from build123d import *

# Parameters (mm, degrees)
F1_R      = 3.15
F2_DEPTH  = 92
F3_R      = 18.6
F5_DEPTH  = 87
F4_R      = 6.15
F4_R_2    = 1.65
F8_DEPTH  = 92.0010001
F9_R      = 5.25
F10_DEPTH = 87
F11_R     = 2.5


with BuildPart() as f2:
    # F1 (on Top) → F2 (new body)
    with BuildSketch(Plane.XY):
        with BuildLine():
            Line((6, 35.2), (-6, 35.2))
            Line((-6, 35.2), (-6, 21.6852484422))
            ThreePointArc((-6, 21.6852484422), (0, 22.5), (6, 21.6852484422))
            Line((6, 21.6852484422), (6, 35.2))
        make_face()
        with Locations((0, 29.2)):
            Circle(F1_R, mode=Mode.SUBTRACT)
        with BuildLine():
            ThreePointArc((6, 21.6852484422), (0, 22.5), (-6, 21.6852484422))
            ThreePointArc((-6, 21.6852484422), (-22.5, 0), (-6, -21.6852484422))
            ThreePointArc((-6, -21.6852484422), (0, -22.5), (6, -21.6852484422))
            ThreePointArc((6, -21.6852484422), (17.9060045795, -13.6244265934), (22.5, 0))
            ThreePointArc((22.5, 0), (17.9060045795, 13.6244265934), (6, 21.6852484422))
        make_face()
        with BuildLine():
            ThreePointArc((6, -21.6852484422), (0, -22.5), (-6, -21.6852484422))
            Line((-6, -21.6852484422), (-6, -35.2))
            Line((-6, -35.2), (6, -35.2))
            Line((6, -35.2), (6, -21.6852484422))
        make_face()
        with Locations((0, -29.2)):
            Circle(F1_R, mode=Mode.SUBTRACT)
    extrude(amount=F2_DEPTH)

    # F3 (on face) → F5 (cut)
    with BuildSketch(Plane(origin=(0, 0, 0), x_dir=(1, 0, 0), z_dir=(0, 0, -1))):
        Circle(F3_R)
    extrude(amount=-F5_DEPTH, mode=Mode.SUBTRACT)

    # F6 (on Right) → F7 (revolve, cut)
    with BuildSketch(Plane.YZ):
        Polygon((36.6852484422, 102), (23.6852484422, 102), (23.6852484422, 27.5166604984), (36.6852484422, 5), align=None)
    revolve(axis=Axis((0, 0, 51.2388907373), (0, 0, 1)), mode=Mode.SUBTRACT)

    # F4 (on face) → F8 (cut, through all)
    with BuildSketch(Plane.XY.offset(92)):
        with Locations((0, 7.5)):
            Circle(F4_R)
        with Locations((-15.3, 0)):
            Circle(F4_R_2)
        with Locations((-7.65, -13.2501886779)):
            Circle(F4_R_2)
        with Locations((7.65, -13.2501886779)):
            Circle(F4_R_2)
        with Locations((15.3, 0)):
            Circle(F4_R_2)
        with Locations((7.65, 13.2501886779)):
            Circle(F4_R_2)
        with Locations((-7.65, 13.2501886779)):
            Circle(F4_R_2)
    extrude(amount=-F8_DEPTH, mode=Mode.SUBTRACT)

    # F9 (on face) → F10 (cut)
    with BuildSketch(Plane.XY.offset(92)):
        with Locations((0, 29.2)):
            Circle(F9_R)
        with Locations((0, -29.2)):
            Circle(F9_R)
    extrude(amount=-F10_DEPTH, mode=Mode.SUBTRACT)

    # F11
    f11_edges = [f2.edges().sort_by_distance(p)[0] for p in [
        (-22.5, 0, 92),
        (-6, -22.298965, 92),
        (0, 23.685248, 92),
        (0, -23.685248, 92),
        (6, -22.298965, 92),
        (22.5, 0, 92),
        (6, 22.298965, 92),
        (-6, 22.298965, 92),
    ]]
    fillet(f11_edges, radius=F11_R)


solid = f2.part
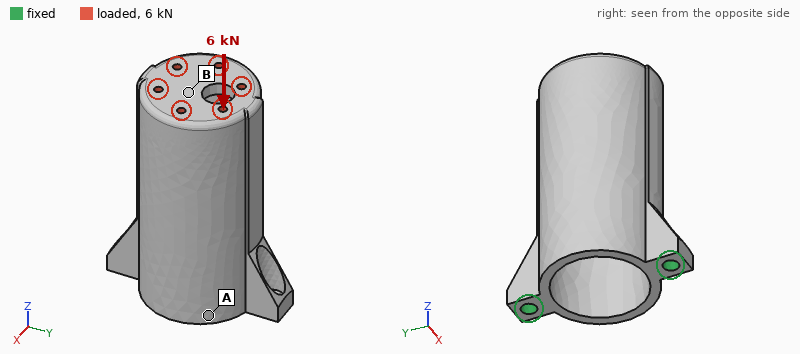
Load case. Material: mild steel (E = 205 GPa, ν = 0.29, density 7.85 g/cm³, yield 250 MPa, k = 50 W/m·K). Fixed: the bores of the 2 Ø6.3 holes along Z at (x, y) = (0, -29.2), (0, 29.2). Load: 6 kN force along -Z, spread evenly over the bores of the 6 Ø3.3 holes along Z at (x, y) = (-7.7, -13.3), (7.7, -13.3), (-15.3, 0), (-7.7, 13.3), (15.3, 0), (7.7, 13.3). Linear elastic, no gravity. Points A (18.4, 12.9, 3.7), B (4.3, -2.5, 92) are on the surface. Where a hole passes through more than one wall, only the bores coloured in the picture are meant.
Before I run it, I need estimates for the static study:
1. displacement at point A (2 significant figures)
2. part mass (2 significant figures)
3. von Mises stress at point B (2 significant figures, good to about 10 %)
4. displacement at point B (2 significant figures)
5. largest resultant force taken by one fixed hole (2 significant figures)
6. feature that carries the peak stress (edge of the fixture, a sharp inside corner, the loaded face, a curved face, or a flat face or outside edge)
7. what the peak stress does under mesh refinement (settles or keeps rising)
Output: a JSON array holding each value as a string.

["8.1 µm", "440 g", "29 MPa", "19 µm", "3.1 kN", "edge of the fixture", "keeps rising"]
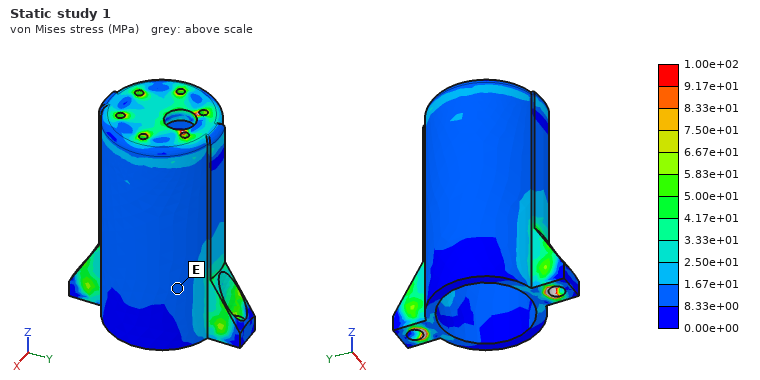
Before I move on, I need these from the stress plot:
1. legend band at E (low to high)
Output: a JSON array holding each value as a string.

["8.33e+00 to 1.67e+01 MPa"]
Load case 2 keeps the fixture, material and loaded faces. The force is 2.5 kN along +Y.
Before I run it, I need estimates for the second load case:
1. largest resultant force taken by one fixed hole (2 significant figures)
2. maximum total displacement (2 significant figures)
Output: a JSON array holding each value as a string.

["4.3 kN", "47 µm"]
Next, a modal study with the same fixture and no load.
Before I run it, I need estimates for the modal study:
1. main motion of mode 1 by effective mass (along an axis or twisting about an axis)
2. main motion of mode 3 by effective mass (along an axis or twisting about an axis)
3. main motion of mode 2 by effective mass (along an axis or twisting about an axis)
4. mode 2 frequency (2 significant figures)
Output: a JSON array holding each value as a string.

["along X", "twisting about Z", "along Y", "3000 Hz"]
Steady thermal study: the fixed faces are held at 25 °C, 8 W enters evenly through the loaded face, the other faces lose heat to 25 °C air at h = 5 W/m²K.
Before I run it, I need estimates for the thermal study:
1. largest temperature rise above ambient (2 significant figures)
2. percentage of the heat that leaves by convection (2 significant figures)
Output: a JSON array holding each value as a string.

["29 K", "28 %"]
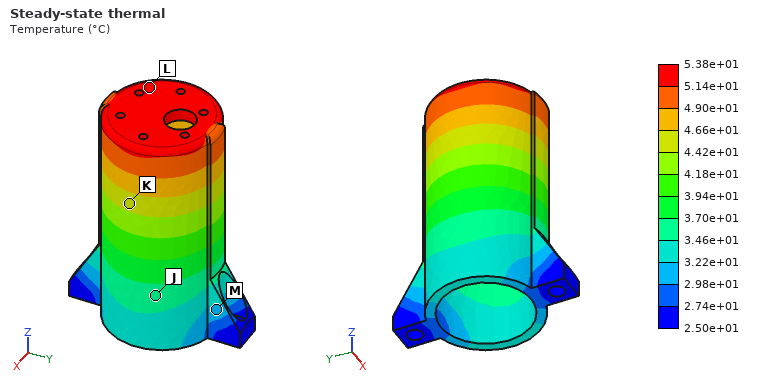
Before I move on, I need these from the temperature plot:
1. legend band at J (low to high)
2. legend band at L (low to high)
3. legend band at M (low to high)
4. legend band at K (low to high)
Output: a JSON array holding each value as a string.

["3.46e+01 to 3.70e+01 °C", "5.14e+01 to 5.38e+01 °C", "2.98e+01 to 3.22e+01 °C", "4.42e+01 to 4.66e+01 °C"]
